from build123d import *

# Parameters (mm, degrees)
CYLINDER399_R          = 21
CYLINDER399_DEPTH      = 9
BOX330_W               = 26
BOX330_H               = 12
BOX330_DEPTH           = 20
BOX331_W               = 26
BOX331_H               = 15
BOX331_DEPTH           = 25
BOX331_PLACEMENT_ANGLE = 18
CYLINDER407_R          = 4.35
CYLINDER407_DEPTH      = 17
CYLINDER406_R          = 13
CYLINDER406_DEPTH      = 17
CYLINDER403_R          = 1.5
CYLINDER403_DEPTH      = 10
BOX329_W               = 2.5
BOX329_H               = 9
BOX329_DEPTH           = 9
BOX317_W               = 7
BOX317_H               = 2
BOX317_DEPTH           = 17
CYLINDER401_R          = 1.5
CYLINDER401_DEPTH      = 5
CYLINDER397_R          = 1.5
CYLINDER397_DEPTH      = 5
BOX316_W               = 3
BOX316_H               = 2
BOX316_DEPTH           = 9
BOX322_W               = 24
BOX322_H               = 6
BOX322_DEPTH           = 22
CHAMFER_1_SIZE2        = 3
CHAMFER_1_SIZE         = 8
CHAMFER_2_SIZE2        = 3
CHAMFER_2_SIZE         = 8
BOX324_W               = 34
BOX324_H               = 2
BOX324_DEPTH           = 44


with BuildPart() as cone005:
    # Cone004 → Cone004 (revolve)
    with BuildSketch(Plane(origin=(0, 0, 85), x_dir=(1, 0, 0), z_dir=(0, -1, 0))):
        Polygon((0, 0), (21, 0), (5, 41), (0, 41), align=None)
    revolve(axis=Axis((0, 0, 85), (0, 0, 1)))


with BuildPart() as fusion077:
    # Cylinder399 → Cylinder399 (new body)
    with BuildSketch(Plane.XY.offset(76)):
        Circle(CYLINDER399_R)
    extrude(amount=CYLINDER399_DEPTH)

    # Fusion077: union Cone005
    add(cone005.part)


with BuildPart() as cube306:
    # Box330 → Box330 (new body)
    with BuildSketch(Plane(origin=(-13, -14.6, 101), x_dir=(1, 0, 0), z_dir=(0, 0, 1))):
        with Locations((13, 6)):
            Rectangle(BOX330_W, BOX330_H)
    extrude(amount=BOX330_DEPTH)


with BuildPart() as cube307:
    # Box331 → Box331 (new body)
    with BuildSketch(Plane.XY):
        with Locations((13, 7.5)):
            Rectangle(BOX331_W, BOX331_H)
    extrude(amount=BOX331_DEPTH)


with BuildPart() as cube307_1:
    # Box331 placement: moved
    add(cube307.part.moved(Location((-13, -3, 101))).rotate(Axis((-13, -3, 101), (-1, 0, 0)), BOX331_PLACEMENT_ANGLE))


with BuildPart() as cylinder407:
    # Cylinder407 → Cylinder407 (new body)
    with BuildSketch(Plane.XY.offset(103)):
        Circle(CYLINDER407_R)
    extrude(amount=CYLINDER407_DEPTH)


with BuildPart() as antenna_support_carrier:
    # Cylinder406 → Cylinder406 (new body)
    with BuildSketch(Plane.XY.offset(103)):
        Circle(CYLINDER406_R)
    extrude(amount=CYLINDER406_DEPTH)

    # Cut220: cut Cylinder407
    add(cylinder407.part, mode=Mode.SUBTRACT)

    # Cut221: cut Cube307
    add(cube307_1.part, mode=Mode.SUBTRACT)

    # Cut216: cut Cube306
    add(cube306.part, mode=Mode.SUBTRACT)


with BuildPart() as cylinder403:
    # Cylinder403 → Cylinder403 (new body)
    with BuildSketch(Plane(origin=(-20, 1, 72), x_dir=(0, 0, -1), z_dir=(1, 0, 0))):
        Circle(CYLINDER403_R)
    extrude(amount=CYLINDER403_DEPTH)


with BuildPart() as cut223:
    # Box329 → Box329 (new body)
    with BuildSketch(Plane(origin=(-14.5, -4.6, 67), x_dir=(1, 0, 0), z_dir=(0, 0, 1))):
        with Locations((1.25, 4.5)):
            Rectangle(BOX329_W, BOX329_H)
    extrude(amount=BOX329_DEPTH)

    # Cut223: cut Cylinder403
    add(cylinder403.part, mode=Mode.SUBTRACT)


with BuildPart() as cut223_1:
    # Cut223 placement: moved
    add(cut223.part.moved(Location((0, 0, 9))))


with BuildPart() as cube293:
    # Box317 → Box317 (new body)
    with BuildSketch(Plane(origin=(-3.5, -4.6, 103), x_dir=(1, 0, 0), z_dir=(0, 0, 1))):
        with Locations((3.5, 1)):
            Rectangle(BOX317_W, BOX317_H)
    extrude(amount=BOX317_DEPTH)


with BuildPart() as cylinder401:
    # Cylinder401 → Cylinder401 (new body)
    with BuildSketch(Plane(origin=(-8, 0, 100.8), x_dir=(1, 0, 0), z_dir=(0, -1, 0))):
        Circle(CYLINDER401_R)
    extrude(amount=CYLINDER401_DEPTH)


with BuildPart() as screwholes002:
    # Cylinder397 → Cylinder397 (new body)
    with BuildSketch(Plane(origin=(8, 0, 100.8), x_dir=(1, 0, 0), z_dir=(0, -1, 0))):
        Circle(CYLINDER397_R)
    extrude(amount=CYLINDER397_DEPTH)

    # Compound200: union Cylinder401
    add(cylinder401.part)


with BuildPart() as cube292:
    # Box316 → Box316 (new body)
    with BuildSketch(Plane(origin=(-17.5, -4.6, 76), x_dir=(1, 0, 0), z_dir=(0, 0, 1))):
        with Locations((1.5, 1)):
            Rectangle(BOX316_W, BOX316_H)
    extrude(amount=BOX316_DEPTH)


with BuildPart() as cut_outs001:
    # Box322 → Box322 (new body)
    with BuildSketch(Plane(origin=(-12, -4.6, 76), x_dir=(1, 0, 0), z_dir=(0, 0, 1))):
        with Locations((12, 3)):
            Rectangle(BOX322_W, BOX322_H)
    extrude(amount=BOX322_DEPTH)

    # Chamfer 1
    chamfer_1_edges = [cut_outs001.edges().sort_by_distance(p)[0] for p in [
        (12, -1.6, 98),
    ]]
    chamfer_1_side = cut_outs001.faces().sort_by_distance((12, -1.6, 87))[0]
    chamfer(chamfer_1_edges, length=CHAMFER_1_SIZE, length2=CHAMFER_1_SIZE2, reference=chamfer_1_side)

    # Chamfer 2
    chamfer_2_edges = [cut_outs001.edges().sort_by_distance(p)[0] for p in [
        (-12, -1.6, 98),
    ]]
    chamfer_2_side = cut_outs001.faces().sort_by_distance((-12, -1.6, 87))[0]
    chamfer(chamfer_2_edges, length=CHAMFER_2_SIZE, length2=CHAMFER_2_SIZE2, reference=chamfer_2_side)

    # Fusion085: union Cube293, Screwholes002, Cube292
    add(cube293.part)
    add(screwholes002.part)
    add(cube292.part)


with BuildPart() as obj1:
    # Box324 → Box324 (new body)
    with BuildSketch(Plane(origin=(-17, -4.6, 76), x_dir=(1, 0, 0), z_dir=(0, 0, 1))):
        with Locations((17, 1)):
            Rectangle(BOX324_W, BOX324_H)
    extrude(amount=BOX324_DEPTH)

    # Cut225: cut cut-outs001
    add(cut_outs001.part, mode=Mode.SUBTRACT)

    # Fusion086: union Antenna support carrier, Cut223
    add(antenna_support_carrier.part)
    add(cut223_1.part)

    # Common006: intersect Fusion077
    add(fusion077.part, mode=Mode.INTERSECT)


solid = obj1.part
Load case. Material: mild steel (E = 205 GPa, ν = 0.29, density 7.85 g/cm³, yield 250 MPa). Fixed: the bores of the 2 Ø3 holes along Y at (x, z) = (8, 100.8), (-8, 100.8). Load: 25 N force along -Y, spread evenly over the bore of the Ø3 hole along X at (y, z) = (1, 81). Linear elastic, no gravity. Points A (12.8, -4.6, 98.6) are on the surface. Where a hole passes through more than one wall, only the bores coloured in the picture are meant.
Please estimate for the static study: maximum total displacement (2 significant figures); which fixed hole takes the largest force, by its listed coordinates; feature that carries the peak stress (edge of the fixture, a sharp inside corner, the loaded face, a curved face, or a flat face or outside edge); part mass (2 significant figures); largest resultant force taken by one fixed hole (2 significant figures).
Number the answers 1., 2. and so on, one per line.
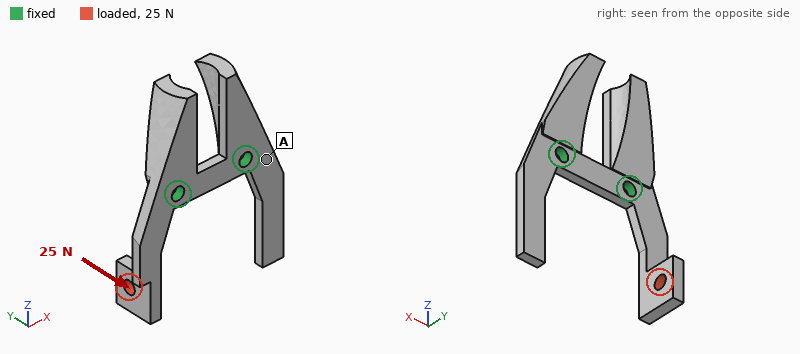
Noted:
1. 0.13 mm
2. (-8, 100.8)
3. a flat face or outside edge
4. 14 g
5. 24 N
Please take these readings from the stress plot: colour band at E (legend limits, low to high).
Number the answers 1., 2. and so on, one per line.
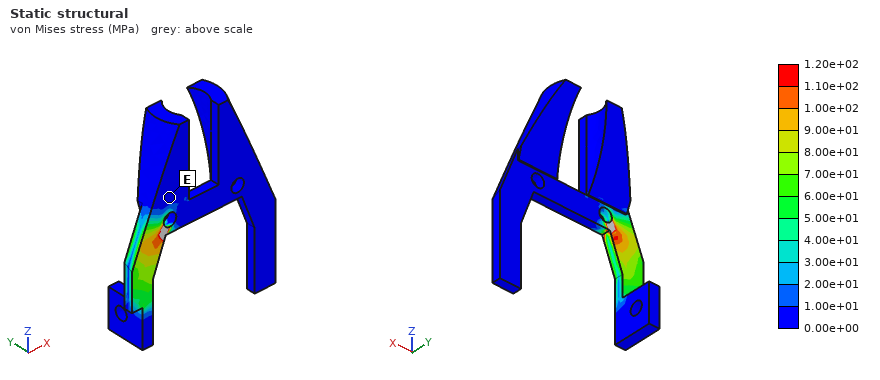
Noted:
1. 0.00e+00 to 1.00e+01 MPa
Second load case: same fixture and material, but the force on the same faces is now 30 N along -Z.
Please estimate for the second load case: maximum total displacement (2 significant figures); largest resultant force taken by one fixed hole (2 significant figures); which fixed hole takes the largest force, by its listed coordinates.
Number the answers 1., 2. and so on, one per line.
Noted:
1. 63 µm
2. 32 N
3. (-8, 100.8)
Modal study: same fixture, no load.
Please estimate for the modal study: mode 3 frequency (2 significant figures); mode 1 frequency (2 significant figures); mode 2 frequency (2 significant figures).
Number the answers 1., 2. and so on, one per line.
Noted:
1. 4100 Hz
2. 1900 Hz
3. 2700 Hz
